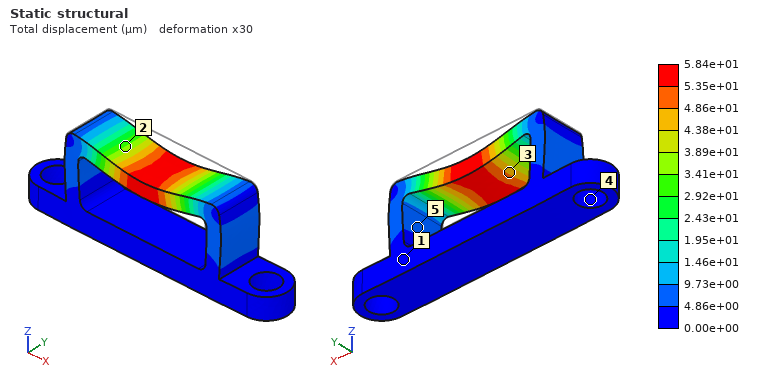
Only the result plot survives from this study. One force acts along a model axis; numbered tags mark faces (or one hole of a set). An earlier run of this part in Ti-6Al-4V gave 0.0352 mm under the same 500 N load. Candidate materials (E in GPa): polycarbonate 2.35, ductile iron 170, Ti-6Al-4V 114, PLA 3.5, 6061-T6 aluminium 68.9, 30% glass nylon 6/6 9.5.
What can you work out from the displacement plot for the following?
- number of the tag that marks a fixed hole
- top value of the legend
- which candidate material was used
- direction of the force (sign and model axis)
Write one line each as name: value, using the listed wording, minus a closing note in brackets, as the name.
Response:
number of the tag that marks a fixed hole: 4
top value of the legend: 5.84e+01 µm
which candidate material was used: 6061-T6 aluminium
direction of the force: -Z
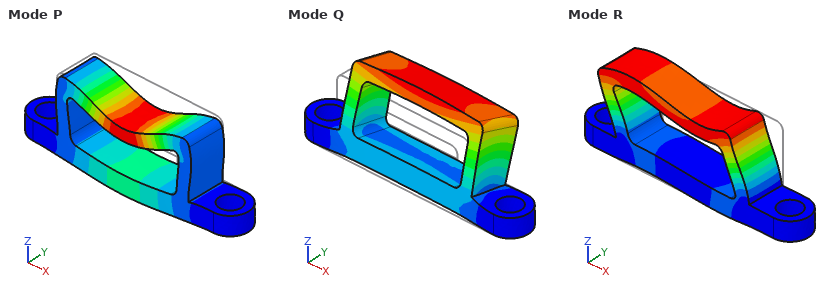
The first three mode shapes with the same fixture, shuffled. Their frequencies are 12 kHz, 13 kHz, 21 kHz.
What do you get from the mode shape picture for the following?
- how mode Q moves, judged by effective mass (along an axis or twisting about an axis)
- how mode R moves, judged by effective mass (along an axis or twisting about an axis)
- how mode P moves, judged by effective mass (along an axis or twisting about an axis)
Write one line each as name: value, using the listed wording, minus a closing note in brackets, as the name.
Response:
how mode Q moves, judged by effective mass: along Y
how mode R moves, judged by effective mass: along X
how mode P moves, judged by effective mass: along Z
